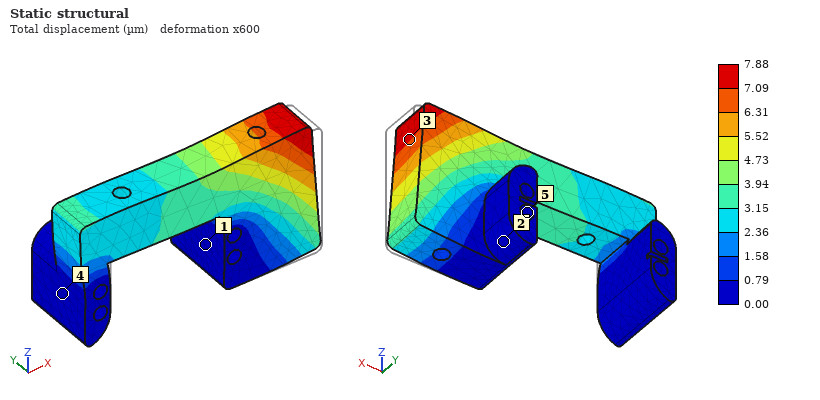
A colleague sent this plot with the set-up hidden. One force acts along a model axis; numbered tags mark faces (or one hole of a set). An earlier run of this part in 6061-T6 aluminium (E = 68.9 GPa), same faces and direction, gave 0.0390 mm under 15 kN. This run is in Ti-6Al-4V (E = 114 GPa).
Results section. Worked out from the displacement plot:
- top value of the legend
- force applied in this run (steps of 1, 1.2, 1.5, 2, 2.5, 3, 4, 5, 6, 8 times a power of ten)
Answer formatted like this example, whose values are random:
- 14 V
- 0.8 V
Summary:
- 7.88 µm
- 5 kN
